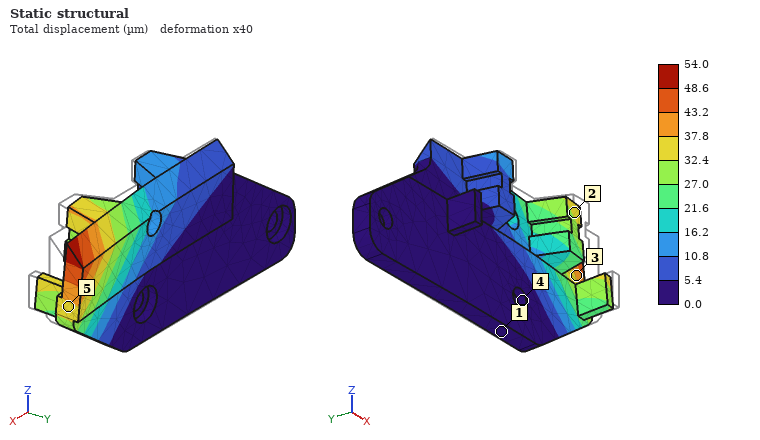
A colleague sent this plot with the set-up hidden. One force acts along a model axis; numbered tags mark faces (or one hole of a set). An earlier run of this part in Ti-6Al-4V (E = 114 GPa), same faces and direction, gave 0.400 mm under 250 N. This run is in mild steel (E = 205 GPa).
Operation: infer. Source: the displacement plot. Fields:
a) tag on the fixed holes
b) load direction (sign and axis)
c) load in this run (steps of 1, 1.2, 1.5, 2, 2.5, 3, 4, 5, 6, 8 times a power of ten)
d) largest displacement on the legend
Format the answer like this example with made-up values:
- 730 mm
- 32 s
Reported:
- 4
- +Y
- 60 N
- 54.0 µm
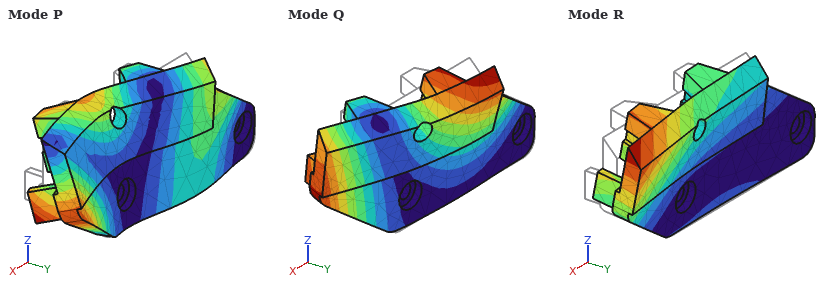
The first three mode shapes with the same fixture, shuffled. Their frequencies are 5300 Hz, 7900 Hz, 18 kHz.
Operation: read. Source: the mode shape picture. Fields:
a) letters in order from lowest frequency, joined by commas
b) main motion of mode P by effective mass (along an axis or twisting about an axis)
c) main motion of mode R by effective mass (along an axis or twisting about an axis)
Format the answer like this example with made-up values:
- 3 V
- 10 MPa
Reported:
- R, Q, P
- along Y
- along Y
